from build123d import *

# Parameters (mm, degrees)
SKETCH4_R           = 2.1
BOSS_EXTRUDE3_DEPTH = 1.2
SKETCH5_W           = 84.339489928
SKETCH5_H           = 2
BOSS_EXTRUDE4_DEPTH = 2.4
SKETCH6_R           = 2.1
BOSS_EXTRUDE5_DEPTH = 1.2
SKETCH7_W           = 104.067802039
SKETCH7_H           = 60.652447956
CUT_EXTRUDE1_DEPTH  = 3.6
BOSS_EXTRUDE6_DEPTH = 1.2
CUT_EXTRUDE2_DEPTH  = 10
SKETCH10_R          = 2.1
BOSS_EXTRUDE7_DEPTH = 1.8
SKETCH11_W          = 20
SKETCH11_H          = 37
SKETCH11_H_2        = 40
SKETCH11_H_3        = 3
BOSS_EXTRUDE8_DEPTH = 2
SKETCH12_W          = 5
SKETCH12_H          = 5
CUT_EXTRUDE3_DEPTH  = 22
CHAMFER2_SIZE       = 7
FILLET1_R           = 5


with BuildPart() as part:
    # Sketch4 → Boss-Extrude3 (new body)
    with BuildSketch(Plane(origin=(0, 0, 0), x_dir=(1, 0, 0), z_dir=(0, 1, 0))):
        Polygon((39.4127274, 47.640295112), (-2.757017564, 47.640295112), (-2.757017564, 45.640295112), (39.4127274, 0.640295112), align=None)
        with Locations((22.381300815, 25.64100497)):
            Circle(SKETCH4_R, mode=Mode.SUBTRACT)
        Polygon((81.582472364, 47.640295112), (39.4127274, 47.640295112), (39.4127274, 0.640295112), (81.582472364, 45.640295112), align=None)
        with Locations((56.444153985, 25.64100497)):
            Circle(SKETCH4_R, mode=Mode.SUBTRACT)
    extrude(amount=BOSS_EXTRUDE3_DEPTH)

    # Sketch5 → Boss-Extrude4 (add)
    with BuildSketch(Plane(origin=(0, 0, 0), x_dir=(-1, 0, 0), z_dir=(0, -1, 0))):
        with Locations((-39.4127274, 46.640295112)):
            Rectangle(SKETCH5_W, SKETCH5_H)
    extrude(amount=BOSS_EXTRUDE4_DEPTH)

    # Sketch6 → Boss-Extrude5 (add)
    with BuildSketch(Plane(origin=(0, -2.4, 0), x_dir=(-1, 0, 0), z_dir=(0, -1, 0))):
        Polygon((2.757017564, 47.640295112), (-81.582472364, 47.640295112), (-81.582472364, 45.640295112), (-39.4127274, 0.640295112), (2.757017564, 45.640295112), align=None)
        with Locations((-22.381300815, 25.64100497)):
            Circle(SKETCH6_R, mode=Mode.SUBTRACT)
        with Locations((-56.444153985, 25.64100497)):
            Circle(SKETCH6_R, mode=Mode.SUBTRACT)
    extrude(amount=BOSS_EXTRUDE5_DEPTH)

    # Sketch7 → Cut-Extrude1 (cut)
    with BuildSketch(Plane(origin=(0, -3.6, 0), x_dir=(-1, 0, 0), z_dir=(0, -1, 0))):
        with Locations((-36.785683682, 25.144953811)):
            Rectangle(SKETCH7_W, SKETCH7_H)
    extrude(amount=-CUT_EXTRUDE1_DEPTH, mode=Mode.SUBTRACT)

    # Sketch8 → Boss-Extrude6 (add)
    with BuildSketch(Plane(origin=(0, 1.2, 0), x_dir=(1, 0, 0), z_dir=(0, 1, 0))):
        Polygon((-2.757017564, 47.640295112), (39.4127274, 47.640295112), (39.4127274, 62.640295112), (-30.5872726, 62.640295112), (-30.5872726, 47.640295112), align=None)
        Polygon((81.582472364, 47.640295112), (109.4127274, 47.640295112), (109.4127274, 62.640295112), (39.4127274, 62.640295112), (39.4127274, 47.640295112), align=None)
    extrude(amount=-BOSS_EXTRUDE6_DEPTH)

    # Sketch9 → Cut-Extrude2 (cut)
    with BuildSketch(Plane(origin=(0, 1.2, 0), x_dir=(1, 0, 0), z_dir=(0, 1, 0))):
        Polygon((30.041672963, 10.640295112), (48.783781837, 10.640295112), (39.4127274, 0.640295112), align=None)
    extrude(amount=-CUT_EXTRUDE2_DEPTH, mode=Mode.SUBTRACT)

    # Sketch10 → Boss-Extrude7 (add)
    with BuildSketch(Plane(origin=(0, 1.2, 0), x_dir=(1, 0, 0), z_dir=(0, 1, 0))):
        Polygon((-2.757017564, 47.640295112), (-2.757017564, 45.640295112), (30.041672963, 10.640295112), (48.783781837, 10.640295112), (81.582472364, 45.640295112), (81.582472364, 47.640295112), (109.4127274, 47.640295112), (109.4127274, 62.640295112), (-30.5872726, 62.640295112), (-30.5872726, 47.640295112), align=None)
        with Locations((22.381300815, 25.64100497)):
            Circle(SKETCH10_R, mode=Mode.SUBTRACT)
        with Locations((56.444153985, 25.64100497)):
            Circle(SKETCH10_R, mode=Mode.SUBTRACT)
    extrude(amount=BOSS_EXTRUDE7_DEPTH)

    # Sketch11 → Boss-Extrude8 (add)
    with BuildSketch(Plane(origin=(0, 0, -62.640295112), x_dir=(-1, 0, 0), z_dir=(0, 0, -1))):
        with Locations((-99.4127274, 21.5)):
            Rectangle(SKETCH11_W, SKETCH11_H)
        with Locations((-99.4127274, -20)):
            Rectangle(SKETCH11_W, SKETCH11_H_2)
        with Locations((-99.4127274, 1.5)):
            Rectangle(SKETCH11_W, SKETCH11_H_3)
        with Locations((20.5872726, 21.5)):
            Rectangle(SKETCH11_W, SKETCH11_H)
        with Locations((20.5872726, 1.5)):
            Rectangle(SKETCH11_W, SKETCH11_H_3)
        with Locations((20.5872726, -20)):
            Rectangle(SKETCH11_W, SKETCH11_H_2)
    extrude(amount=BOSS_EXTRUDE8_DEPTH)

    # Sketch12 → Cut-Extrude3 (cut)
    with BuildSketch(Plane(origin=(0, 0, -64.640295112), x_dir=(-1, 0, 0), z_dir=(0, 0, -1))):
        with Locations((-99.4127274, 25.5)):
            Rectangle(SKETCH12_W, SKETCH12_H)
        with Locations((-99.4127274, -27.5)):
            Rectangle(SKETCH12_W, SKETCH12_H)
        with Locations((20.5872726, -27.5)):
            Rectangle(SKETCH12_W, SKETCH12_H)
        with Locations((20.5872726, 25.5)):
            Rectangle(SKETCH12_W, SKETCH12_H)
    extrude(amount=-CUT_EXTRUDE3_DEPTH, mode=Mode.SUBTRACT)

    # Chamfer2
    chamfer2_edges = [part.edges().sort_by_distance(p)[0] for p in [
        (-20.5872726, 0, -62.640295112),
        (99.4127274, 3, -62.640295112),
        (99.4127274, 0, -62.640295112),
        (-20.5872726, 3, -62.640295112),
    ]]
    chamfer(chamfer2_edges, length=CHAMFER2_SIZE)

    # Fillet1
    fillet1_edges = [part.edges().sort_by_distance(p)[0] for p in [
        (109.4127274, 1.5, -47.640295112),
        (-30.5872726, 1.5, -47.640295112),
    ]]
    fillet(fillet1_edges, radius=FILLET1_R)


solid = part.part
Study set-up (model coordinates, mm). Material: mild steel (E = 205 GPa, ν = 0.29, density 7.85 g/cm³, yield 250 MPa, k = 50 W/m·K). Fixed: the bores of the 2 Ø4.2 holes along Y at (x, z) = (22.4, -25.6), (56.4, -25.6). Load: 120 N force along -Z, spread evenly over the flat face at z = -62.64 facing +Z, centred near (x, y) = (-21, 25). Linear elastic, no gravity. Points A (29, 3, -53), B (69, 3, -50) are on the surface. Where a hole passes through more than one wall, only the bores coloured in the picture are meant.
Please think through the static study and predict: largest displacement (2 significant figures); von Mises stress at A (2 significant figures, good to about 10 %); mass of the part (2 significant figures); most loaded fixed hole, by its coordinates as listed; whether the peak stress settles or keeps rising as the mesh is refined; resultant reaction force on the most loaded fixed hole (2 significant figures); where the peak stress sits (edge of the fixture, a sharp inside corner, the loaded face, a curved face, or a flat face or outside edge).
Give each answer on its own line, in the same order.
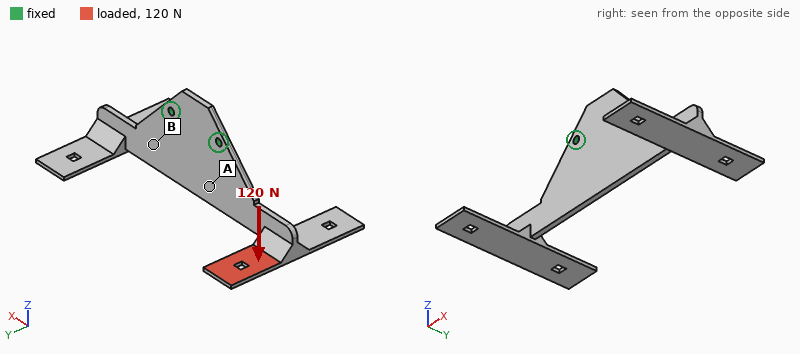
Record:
0.63 mm
31 MPa
160 g
(22.4, -25.6)
keeps rising
270 N
a sharp inside corner
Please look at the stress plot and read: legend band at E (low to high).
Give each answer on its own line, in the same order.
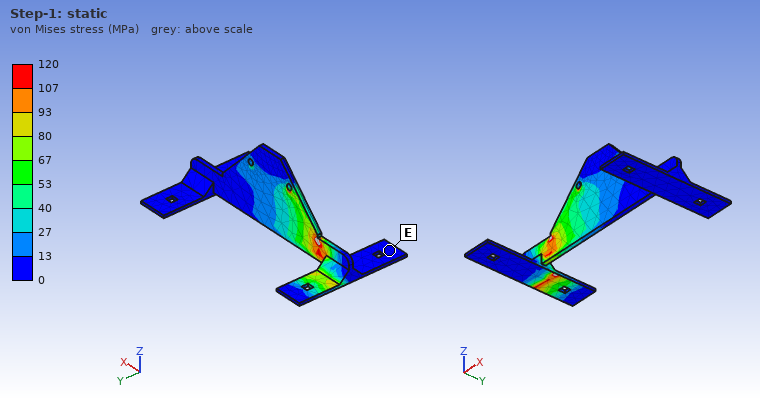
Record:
0 to 13 MPa
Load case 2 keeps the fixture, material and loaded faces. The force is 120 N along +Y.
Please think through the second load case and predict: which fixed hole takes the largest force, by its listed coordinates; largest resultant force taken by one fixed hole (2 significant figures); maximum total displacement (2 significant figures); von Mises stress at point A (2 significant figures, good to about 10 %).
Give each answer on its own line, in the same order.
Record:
(22.4, -25.6)
220 N
0.99 mm
72 MPa
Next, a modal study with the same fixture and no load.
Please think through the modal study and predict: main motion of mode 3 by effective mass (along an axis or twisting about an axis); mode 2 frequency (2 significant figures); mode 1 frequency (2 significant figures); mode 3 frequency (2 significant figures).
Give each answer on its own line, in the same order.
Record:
twisting about X
320 Hz
320 Hz
640 Hz
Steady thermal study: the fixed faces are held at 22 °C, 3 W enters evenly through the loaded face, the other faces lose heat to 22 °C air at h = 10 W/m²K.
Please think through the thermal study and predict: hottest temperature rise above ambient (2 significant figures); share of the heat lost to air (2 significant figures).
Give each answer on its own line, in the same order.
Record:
55 K
50 %
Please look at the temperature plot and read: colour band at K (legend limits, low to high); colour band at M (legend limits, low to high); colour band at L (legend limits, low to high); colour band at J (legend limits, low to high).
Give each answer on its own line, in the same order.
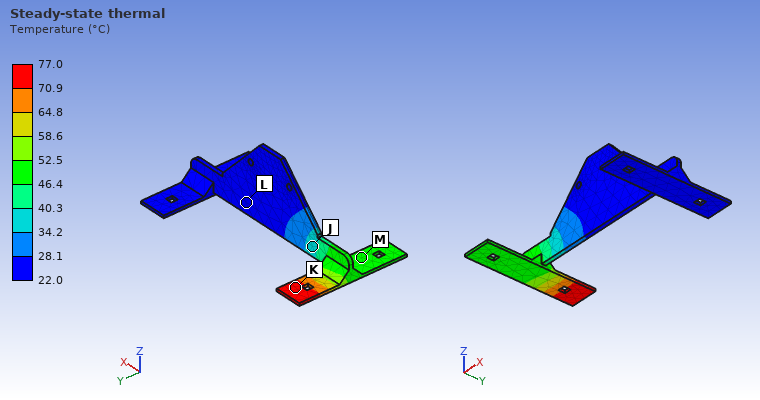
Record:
70.9 to 77.0 °C
46.4 to 52.5 °C
22.0 to 28.1 °C
34.2 to 40.3 °C
